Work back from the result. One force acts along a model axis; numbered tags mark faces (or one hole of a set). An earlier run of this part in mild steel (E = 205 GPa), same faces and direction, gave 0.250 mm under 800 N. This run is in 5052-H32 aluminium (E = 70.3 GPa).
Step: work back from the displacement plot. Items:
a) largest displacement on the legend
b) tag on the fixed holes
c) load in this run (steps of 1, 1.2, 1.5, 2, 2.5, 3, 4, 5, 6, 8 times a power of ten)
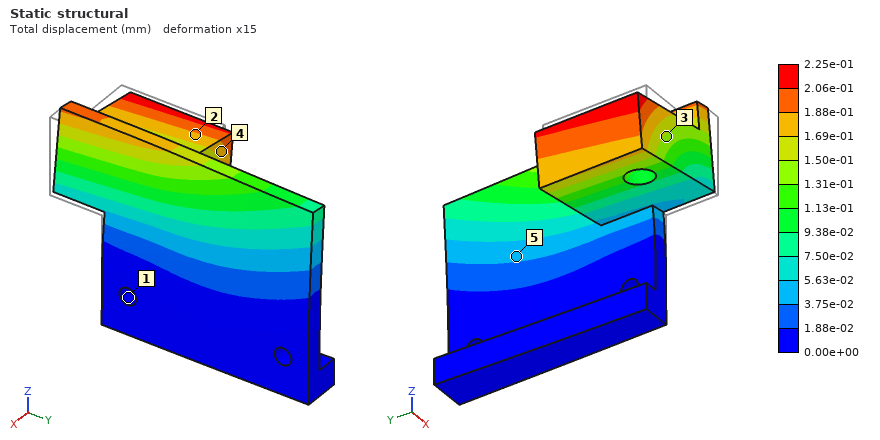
2.25e-01 mm
1
250 N
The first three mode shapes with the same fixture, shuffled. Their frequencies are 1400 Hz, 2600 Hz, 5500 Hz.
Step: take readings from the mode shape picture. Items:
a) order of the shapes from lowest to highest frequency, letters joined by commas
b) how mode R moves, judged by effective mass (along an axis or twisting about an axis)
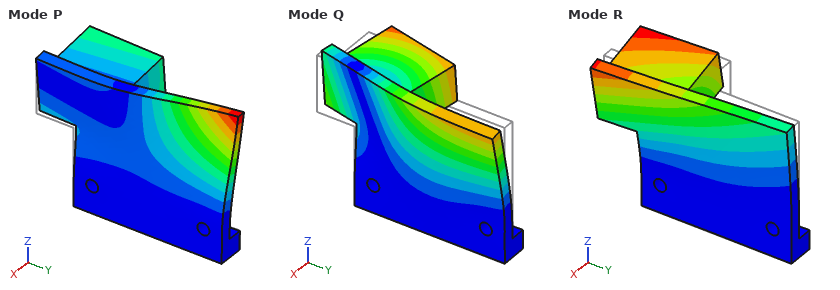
R, Q, P
along X
